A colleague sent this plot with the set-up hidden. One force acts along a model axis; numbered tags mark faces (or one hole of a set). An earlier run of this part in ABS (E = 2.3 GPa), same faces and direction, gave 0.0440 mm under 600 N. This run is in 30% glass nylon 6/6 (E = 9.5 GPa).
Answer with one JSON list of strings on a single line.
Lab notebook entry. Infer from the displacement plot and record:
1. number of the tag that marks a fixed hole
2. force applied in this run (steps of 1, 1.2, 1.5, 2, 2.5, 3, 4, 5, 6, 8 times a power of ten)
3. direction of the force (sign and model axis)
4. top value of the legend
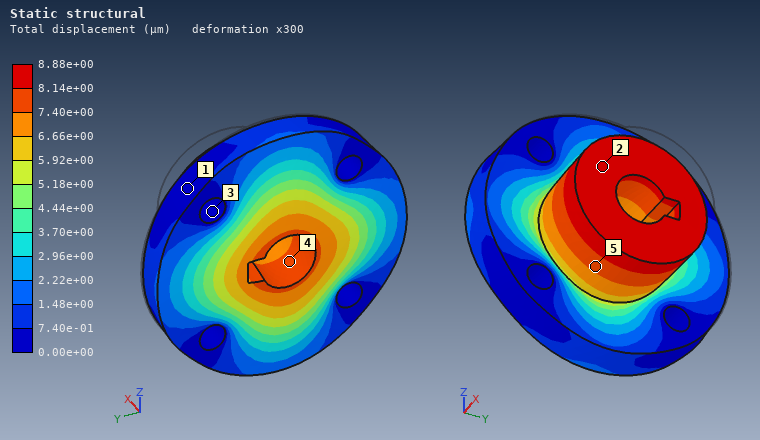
["3", "500 N", "-X", "8.88e+00 µm"]
